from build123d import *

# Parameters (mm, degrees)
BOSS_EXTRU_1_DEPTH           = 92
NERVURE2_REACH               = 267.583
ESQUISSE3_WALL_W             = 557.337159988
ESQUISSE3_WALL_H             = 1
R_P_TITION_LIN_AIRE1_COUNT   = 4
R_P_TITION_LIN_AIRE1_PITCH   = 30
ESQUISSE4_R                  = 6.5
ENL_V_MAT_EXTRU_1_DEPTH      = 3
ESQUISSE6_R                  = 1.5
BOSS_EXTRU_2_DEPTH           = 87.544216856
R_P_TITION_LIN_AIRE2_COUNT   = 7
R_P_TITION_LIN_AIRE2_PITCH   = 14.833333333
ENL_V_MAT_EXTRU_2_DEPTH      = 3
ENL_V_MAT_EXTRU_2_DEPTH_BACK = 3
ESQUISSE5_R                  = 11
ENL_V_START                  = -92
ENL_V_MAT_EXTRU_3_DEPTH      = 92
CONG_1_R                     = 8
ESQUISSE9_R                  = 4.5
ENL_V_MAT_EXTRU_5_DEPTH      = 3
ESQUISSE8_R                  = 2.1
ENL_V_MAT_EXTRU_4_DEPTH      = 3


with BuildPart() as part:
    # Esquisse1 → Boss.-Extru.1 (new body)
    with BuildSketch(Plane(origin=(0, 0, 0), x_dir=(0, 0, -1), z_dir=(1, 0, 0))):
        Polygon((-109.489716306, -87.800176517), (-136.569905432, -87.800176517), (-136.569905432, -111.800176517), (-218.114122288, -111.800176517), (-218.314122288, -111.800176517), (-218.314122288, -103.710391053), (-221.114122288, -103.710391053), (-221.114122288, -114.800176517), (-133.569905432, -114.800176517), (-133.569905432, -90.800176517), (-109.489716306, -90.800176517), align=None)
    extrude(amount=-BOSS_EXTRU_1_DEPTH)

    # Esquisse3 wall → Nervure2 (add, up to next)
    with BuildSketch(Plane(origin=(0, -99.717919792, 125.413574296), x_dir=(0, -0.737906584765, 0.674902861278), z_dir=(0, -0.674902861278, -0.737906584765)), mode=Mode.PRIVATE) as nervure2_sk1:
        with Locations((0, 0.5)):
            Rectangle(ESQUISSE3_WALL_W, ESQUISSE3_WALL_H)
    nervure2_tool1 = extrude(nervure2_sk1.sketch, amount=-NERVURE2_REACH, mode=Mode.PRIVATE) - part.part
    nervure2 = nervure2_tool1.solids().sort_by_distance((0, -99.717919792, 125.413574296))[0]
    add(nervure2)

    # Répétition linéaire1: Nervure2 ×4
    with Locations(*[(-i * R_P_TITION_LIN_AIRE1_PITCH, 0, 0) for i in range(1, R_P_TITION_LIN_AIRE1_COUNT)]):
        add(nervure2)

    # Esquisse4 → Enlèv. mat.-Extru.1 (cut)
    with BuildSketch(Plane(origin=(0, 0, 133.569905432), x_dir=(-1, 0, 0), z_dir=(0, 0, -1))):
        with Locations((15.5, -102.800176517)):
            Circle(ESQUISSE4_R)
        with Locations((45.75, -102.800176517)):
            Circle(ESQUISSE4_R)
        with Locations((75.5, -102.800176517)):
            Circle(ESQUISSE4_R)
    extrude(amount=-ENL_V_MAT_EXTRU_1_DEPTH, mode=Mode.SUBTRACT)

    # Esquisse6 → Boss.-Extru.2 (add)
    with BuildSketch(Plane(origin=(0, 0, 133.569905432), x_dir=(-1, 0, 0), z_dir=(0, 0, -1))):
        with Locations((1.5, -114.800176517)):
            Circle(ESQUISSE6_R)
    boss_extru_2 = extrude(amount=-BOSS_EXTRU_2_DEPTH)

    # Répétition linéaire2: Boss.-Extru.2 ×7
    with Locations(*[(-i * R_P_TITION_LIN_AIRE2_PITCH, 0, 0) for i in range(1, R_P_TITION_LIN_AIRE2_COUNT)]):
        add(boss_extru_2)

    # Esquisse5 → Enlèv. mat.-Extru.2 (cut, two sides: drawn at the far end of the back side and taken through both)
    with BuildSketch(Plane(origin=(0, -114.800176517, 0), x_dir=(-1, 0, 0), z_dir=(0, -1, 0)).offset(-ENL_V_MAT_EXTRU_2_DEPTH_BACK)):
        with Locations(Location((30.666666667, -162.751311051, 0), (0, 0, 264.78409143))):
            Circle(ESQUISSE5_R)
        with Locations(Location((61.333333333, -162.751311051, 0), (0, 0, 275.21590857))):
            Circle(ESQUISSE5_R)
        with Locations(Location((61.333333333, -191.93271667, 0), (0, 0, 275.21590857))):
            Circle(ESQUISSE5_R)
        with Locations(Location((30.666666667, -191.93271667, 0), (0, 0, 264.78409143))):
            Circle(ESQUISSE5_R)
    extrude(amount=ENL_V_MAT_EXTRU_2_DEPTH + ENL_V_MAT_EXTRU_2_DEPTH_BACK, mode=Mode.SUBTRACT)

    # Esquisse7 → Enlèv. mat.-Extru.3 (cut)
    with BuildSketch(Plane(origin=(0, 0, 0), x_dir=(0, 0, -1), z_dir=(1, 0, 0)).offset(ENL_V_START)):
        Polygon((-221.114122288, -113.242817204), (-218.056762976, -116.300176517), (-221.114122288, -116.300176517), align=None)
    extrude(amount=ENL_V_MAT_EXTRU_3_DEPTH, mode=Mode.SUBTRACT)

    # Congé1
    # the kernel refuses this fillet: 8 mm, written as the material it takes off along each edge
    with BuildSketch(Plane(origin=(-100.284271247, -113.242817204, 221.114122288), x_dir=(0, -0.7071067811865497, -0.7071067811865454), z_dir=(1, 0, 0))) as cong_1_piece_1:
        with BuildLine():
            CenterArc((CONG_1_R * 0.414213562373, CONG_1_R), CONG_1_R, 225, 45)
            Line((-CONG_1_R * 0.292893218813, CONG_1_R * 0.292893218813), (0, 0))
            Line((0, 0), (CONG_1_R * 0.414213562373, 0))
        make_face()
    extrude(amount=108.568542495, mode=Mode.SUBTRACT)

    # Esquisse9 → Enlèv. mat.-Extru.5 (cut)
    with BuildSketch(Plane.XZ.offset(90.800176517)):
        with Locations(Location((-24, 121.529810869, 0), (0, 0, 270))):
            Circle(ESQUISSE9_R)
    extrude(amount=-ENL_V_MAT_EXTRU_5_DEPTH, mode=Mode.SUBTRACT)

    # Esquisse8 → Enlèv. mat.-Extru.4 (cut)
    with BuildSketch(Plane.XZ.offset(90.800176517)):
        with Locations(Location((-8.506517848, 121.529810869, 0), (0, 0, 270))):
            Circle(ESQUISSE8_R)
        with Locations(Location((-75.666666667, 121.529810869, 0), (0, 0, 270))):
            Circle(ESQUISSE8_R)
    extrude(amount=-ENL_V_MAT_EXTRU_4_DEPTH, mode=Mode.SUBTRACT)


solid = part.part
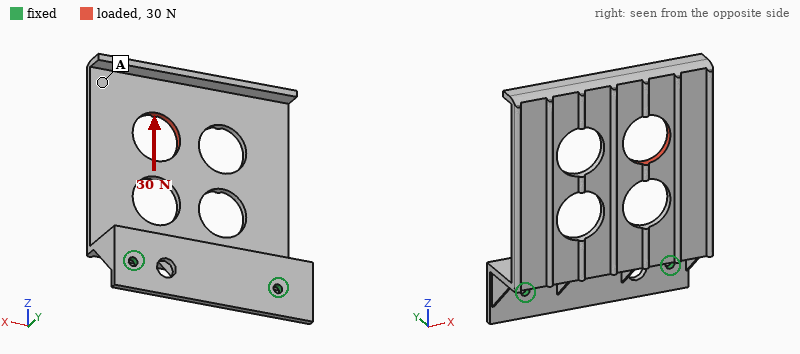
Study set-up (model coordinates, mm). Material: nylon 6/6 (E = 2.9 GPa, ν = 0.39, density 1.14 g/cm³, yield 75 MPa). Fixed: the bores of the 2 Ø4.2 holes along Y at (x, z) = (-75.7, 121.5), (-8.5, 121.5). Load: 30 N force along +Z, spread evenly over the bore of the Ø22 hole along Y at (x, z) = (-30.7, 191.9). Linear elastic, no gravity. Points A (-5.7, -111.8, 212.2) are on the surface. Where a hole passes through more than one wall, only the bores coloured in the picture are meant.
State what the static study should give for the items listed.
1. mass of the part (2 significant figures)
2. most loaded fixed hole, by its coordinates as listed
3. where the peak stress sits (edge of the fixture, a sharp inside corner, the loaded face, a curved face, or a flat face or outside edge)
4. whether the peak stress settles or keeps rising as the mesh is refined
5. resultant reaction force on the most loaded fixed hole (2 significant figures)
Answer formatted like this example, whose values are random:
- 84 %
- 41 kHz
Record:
- 41 g
- (-8.5, 121.5)
- edge of the fixture
- keeps rising
- 20 N
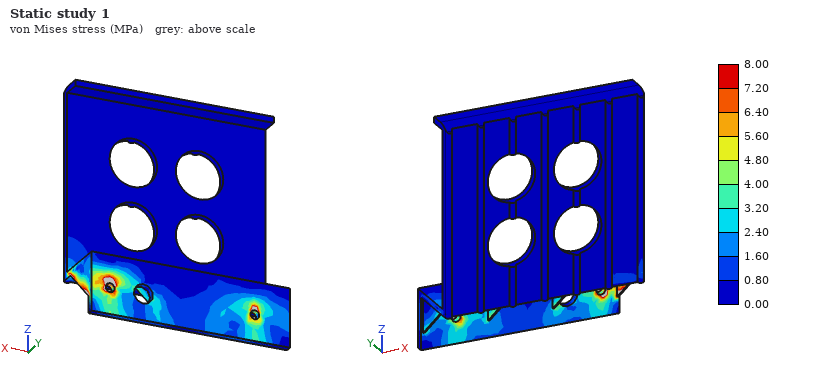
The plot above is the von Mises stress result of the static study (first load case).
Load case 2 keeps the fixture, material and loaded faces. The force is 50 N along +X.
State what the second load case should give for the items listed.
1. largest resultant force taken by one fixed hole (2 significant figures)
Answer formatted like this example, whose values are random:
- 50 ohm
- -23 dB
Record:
- 58 N
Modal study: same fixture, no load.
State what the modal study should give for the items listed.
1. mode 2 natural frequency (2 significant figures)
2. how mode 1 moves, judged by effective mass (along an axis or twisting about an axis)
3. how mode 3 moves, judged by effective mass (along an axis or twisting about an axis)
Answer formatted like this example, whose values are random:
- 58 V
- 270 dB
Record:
- 170 Hz
- along Y
- along X
